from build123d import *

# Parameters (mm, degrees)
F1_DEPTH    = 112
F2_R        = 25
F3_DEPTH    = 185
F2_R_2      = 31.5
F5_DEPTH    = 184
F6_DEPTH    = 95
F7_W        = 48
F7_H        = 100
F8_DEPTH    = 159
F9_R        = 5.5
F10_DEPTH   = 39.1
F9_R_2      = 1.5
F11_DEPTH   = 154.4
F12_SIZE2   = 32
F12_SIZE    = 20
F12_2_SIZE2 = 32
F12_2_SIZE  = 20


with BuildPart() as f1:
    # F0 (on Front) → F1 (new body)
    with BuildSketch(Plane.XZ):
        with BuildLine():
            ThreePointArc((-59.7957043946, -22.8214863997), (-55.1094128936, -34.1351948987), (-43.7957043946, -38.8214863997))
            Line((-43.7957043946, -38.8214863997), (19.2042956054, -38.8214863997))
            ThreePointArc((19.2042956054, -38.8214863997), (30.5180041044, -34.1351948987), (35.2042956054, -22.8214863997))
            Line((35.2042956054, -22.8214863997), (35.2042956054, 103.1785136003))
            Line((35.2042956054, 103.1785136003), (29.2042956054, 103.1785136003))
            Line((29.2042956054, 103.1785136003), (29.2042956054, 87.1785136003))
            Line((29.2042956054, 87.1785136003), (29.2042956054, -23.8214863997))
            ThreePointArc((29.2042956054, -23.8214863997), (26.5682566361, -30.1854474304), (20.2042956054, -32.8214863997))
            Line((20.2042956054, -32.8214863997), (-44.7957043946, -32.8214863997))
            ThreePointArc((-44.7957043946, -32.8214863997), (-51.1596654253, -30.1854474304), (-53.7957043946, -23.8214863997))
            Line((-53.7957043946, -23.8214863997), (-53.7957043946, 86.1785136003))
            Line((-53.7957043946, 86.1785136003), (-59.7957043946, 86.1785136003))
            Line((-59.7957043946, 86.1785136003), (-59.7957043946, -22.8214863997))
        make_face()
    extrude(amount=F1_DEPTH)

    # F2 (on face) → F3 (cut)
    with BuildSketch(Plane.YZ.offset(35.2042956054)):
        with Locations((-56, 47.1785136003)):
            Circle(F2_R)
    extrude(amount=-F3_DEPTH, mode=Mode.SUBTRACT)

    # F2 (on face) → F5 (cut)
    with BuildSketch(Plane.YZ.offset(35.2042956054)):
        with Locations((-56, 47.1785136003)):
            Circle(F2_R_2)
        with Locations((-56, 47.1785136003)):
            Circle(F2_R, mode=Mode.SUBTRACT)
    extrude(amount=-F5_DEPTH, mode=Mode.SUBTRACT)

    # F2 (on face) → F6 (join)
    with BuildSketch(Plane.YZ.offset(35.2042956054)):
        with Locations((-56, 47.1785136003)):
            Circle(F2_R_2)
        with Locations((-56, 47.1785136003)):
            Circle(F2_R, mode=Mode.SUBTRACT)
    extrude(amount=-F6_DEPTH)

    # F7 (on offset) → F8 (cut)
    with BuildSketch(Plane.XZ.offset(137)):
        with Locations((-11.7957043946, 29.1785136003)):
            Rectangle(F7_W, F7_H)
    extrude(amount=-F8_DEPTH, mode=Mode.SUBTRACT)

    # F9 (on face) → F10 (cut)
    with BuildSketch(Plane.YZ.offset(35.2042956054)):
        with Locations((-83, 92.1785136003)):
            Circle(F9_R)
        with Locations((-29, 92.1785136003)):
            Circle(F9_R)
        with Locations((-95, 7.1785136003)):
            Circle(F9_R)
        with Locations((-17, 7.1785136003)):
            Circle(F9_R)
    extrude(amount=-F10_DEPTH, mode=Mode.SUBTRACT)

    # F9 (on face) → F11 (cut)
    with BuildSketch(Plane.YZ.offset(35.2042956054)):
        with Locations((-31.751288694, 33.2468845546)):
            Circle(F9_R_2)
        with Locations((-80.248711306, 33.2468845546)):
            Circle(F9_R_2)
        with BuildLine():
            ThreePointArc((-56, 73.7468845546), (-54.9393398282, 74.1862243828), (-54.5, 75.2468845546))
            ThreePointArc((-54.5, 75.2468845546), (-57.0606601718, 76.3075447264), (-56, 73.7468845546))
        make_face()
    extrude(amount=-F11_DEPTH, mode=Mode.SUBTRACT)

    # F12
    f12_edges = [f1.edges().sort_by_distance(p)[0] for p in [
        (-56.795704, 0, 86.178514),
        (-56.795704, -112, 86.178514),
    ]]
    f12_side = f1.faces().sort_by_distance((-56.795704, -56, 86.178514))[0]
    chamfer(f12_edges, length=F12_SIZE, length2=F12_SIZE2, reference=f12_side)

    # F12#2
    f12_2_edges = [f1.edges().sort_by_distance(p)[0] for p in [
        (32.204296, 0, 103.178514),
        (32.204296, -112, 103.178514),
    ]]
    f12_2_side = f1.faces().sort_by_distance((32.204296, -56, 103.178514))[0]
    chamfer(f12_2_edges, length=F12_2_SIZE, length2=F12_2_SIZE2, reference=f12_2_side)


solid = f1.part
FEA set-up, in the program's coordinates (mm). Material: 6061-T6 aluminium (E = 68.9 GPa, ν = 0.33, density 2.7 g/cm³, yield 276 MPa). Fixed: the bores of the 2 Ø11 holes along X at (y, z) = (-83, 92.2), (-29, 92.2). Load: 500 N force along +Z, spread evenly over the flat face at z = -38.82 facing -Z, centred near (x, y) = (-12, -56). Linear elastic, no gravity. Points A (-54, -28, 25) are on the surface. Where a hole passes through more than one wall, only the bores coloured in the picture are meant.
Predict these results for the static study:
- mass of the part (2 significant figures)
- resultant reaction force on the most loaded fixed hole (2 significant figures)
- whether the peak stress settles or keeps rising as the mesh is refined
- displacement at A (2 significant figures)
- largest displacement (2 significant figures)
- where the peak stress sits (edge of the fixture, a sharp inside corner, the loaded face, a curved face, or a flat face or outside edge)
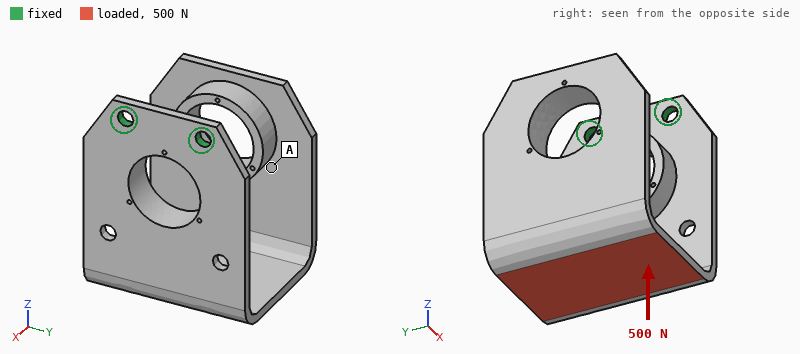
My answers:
630 g
280 N
keeps rising
1.6 mm
2.2 mm
edge of the fixture
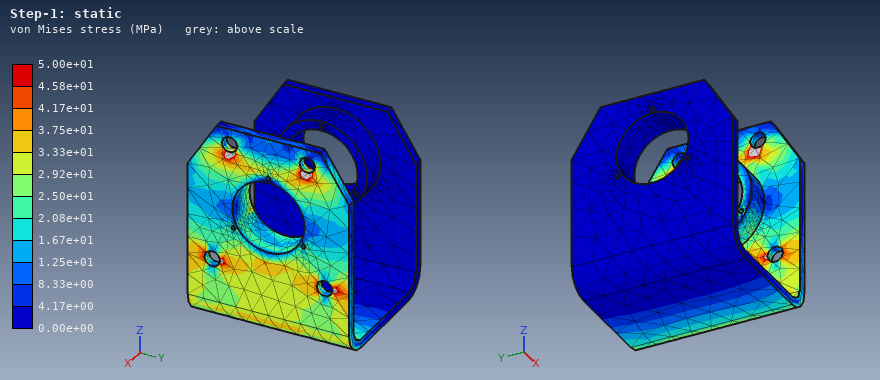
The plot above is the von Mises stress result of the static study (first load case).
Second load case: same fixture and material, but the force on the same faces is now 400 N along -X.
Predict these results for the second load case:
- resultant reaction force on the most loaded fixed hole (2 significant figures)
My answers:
360 N
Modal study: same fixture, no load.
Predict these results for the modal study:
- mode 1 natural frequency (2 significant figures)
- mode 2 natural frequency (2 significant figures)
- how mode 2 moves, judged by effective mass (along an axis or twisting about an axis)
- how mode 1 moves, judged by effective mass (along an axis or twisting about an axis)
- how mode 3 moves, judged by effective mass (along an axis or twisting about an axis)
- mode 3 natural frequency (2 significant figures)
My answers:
99 Hz
140 Hz
along Y
along Z
along X
150 Hz
